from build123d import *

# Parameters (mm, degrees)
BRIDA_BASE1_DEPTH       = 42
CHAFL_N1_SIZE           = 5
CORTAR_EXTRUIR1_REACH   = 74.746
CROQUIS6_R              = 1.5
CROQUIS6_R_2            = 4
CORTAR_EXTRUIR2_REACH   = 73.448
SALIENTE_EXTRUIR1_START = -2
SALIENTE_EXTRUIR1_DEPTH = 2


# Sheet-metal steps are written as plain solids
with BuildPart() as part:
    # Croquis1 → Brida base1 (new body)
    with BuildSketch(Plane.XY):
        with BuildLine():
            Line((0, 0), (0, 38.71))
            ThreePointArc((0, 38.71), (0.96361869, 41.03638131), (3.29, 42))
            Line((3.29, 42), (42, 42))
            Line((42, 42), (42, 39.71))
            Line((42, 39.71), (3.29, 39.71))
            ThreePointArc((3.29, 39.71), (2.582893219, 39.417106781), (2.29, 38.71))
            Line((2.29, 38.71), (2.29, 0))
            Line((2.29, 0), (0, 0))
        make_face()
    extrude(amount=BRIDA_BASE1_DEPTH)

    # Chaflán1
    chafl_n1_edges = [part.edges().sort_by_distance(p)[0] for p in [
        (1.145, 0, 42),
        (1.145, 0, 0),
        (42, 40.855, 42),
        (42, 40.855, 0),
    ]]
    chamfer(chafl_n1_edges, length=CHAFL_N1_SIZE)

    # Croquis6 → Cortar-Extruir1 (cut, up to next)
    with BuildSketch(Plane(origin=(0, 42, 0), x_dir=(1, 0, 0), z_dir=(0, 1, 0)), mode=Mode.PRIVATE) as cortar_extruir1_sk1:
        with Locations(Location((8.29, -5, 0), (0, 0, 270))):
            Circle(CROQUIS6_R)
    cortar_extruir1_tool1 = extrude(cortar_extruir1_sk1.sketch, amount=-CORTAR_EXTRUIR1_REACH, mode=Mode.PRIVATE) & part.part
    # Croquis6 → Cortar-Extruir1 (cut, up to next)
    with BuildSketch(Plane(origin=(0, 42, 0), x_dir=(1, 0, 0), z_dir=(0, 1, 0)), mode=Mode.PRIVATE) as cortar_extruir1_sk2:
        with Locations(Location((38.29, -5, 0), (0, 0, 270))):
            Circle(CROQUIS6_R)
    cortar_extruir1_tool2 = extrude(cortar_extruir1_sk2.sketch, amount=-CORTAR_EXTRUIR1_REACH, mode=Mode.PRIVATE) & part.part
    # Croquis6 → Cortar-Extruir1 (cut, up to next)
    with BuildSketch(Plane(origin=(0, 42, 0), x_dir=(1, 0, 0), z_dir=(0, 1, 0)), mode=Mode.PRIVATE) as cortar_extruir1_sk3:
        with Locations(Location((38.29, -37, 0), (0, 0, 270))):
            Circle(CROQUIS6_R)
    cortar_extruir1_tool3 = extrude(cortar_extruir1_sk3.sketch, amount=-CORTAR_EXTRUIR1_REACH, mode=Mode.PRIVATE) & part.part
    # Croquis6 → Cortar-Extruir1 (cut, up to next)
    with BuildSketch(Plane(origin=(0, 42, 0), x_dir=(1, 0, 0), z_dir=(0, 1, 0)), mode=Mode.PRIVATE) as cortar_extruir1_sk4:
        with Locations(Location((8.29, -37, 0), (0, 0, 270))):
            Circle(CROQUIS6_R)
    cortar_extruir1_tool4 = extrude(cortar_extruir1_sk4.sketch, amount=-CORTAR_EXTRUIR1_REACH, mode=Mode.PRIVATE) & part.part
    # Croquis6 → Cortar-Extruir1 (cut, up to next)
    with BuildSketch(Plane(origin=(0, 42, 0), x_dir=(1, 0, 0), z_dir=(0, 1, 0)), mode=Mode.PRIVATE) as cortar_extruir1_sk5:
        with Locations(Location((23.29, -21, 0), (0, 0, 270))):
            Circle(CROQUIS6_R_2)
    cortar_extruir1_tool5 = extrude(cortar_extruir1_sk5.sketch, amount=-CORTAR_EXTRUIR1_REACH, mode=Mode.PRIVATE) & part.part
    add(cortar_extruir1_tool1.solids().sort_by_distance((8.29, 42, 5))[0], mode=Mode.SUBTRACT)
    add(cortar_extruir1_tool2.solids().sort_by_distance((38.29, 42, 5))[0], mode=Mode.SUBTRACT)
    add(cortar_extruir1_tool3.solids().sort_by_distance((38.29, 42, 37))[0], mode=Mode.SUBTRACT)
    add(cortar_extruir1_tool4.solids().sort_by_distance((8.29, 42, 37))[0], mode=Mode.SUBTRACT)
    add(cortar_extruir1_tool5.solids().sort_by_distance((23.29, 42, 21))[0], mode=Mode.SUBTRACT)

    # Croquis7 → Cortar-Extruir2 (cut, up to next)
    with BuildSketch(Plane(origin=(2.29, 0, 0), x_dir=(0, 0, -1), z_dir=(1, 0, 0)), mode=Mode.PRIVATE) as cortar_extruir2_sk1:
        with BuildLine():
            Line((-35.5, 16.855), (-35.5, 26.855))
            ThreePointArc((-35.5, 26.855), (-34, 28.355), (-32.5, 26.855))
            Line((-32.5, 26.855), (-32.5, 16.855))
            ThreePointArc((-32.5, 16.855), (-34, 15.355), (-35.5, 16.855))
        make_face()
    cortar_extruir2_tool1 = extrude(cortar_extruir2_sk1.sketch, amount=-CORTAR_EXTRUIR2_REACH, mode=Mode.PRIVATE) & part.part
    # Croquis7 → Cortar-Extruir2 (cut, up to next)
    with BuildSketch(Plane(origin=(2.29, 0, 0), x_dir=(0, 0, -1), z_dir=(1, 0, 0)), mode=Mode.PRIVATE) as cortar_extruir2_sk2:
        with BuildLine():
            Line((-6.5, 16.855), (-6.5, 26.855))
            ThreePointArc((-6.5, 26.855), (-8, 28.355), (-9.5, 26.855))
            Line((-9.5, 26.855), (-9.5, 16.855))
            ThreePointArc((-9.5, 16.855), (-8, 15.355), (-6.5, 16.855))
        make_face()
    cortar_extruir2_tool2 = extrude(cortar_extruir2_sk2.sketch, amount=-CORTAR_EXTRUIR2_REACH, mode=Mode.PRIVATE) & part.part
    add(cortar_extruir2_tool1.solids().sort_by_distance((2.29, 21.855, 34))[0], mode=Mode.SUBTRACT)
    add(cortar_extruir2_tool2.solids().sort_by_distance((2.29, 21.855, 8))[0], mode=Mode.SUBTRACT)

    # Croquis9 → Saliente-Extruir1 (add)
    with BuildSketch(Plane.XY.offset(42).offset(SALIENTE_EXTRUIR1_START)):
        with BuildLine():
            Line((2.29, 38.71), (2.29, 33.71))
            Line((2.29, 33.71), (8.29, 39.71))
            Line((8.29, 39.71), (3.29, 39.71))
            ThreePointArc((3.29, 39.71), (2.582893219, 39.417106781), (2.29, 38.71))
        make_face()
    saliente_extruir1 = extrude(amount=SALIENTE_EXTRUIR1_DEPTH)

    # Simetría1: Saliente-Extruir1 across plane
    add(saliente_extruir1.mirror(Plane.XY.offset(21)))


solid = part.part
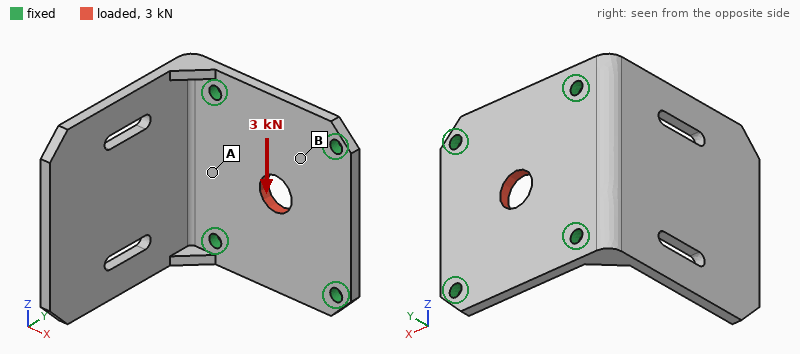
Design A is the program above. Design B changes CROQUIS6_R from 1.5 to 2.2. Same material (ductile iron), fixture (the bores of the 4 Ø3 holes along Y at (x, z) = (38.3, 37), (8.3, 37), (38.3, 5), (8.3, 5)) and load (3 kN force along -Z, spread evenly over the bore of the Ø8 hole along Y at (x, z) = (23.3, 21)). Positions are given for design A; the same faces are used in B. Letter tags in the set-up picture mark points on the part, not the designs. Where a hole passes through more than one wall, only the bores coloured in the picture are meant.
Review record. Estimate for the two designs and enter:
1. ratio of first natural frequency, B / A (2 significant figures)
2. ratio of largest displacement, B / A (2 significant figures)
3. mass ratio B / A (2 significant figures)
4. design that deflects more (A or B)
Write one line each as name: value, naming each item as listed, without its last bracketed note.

ratio of first natural frequency, B / A: 1.0
ratio of largest displacement, B / A: 0.92
mass ratio B / A: 0.99
design that deflects more: A
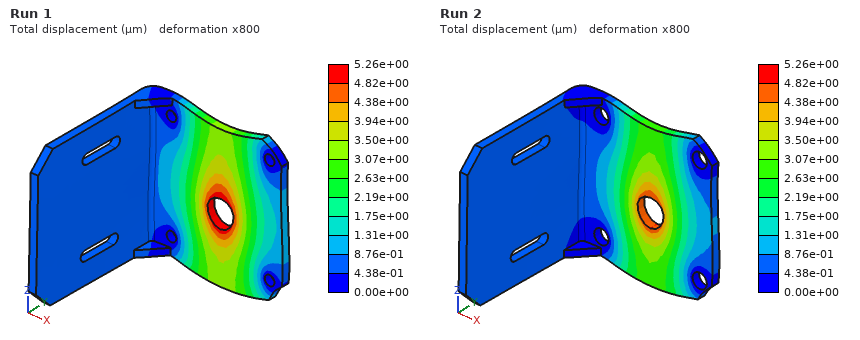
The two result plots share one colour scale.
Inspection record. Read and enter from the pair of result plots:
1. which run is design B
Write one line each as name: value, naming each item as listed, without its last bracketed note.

which run is design B: Run 2
